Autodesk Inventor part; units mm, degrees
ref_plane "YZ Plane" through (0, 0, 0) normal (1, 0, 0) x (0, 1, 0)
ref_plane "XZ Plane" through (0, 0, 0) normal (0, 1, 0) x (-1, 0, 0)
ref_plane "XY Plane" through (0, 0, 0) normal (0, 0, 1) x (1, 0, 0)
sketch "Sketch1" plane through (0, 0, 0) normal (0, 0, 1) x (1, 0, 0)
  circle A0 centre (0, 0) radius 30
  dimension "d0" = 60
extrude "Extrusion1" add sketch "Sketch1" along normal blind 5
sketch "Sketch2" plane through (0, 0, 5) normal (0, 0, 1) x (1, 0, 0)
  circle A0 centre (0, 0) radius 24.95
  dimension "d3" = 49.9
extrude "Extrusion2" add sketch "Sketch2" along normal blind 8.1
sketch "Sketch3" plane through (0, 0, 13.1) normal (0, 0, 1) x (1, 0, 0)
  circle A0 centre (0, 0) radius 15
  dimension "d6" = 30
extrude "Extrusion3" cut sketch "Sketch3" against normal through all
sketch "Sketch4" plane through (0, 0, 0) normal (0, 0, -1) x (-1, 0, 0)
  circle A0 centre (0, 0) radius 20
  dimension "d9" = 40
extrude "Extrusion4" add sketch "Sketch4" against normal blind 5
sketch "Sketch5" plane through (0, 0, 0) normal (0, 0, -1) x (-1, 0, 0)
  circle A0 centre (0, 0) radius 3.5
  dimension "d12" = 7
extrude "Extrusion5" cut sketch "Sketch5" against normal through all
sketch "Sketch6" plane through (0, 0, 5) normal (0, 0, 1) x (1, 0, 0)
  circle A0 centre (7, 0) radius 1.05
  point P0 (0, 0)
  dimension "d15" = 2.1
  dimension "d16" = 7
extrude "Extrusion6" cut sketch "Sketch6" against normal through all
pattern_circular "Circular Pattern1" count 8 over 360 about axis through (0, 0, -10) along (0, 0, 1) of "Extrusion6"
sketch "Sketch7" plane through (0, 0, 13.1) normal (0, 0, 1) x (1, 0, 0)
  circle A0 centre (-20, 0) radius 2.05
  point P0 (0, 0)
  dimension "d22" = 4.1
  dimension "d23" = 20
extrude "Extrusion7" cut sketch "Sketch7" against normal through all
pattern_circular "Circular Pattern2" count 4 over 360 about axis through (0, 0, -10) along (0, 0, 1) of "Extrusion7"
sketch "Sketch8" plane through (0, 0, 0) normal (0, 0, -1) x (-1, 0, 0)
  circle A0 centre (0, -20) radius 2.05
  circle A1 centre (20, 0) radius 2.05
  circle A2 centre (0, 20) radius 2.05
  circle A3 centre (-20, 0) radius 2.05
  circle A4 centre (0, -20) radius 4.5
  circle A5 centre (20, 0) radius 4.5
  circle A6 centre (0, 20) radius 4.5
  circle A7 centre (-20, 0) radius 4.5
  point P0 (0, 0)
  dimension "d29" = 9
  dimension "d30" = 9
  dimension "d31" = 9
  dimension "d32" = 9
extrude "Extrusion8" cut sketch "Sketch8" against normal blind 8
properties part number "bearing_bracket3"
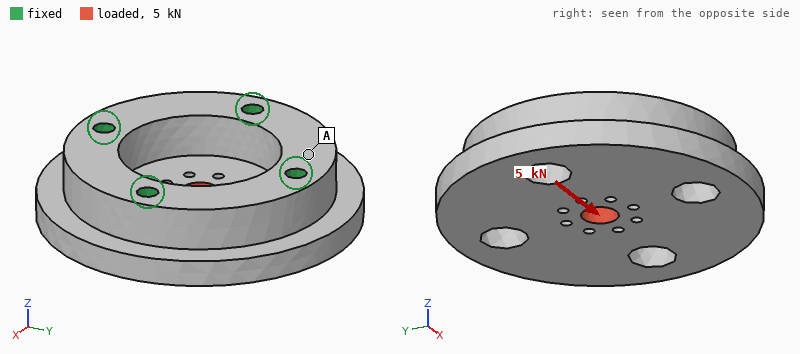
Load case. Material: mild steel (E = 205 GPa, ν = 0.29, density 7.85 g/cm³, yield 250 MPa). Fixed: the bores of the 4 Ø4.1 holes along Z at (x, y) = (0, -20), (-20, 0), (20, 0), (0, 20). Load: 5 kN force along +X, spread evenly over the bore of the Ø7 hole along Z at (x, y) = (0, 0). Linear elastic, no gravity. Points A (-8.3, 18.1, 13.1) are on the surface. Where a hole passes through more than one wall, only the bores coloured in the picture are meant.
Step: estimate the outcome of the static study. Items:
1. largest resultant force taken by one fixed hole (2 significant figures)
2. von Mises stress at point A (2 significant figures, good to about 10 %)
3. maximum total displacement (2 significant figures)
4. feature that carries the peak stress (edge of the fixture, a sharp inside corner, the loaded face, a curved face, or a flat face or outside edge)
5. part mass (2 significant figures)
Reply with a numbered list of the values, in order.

1. 1.5 kN
2. 8.8 MPa
3. 5.4 µm
4. a curved face
5. 170 g
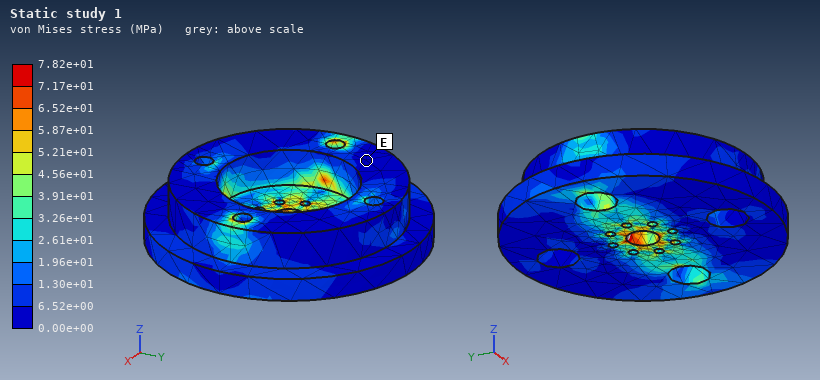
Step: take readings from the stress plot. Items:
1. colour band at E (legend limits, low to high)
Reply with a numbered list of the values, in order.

1. 0.00e+00 to 6.52e+00 MPa
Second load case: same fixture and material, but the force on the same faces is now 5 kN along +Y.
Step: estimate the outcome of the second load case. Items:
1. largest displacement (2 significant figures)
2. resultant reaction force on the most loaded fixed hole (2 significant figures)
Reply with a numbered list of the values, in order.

1. 5.4 µm
2. 1.5 kN
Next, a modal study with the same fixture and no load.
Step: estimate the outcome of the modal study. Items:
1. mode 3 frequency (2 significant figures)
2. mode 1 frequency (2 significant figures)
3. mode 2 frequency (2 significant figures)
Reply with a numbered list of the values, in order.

1. 20 kHz
2. 18 kHz
3. 18 kHz
